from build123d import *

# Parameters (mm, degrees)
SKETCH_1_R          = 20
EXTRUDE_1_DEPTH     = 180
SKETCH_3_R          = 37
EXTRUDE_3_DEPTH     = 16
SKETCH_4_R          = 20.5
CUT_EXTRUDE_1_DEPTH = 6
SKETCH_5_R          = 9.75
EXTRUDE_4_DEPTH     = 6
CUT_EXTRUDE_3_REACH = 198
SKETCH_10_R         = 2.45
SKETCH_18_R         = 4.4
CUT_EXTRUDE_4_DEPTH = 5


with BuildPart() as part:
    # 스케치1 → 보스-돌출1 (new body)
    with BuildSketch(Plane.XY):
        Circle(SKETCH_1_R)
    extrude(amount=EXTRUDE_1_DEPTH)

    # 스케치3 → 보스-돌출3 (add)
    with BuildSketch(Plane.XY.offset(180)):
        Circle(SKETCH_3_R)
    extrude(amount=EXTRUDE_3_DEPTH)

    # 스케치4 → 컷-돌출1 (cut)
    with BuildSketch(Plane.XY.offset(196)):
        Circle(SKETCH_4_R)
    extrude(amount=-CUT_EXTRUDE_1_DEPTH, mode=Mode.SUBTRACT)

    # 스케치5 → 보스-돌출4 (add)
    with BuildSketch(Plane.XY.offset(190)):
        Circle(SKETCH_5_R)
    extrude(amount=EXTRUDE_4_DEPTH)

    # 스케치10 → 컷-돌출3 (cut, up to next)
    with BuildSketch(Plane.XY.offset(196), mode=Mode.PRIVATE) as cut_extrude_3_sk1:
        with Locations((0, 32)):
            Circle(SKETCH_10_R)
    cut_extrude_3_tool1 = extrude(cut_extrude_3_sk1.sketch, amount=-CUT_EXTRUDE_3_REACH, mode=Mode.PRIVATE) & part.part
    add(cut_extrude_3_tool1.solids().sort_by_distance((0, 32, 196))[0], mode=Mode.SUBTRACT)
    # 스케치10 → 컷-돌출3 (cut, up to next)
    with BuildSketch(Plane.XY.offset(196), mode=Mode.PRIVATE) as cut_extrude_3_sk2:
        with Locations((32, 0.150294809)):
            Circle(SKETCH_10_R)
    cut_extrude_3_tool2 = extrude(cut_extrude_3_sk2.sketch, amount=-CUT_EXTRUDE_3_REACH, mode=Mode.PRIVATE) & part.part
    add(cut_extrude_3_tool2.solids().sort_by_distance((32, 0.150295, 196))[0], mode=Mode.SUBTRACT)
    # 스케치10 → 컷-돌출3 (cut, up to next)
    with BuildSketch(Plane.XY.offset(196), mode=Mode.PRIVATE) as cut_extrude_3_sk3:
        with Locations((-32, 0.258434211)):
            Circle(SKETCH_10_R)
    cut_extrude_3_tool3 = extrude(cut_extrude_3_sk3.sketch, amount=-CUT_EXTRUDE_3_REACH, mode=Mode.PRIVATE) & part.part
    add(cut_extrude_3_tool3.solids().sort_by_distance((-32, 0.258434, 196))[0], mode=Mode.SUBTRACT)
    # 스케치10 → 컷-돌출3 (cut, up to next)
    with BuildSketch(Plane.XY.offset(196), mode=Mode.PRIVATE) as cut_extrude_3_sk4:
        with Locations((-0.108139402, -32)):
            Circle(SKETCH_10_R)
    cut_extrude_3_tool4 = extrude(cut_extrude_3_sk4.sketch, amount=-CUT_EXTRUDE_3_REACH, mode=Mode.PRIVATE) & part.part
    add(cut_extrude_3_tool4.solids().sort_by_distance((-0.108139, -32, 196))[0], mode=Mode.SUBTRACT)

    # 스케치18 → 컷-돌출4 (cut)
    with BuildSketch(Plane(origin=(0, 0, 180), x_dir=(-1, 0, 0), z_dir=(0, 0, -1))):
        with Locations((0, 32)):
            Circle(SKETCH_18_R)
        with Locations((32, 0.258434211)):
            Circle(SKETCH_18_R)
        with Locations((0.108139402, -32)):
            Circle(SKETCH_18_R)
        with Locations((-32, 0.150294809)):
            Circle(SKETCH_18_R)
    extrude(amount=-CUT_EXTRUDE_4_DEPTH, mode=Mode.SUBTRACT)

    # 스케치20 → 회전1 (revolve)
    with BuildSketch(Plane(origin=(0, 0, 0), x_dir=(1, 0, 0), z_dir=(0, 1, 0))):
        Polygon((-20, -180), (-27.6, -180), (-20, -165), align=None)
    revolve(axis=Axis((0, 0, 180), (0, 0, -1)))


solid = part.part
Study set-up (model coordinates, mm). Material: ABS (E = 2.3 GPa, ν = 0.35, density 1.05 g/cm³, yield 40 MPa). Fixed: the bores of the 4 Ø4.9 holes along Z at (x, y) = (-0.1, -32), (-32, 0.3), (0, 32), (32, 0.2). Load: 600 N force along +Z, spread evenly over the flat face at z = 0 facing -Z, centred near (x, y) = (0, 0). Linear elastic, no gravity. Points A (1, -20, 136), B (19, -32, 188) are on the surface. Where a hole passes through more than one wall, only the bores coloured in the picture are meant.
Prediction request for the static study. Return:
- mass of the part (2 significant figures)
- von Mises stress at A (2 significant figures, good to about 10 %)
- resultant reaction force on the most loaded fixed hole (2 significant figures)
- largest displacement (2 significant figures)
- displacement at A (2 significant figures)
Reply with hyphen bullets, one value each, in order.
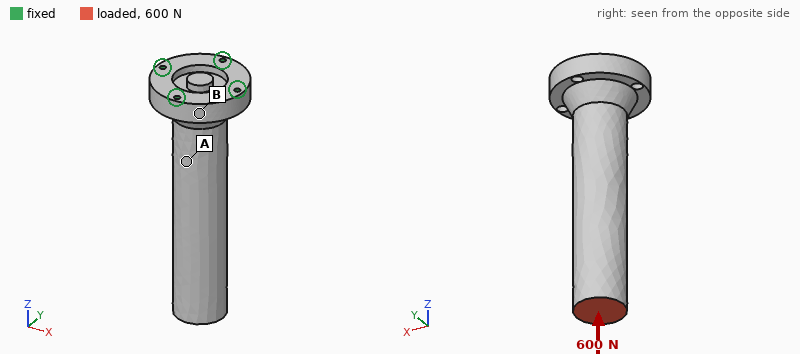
- 310 g
- 0.47 MPa
- 170 N
- 46 µm
- 18 µm
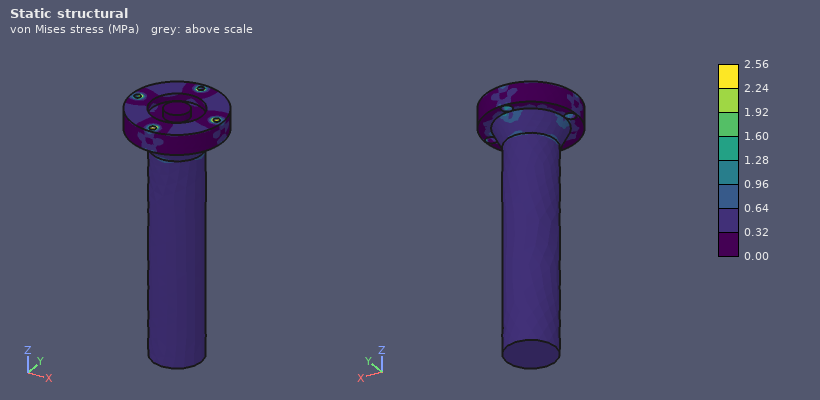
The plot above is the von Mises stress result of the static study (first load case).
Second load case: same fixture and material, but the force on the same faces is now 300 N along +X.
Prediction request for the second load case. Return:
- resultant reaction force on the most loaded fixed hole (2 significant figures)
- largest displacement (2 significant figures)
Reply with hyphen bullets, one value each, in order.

- 940 N
- 2.3 mm
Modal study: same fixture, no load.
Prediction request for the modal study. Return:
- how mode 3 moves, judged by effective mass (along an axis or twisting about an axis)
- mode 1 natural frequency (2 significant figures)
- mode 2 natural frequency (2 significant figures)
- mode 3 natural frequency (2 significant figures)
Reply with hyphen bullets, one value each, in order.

- twisting about Z
- 230 Hz
- 230 Hz
- 1300 Hz
